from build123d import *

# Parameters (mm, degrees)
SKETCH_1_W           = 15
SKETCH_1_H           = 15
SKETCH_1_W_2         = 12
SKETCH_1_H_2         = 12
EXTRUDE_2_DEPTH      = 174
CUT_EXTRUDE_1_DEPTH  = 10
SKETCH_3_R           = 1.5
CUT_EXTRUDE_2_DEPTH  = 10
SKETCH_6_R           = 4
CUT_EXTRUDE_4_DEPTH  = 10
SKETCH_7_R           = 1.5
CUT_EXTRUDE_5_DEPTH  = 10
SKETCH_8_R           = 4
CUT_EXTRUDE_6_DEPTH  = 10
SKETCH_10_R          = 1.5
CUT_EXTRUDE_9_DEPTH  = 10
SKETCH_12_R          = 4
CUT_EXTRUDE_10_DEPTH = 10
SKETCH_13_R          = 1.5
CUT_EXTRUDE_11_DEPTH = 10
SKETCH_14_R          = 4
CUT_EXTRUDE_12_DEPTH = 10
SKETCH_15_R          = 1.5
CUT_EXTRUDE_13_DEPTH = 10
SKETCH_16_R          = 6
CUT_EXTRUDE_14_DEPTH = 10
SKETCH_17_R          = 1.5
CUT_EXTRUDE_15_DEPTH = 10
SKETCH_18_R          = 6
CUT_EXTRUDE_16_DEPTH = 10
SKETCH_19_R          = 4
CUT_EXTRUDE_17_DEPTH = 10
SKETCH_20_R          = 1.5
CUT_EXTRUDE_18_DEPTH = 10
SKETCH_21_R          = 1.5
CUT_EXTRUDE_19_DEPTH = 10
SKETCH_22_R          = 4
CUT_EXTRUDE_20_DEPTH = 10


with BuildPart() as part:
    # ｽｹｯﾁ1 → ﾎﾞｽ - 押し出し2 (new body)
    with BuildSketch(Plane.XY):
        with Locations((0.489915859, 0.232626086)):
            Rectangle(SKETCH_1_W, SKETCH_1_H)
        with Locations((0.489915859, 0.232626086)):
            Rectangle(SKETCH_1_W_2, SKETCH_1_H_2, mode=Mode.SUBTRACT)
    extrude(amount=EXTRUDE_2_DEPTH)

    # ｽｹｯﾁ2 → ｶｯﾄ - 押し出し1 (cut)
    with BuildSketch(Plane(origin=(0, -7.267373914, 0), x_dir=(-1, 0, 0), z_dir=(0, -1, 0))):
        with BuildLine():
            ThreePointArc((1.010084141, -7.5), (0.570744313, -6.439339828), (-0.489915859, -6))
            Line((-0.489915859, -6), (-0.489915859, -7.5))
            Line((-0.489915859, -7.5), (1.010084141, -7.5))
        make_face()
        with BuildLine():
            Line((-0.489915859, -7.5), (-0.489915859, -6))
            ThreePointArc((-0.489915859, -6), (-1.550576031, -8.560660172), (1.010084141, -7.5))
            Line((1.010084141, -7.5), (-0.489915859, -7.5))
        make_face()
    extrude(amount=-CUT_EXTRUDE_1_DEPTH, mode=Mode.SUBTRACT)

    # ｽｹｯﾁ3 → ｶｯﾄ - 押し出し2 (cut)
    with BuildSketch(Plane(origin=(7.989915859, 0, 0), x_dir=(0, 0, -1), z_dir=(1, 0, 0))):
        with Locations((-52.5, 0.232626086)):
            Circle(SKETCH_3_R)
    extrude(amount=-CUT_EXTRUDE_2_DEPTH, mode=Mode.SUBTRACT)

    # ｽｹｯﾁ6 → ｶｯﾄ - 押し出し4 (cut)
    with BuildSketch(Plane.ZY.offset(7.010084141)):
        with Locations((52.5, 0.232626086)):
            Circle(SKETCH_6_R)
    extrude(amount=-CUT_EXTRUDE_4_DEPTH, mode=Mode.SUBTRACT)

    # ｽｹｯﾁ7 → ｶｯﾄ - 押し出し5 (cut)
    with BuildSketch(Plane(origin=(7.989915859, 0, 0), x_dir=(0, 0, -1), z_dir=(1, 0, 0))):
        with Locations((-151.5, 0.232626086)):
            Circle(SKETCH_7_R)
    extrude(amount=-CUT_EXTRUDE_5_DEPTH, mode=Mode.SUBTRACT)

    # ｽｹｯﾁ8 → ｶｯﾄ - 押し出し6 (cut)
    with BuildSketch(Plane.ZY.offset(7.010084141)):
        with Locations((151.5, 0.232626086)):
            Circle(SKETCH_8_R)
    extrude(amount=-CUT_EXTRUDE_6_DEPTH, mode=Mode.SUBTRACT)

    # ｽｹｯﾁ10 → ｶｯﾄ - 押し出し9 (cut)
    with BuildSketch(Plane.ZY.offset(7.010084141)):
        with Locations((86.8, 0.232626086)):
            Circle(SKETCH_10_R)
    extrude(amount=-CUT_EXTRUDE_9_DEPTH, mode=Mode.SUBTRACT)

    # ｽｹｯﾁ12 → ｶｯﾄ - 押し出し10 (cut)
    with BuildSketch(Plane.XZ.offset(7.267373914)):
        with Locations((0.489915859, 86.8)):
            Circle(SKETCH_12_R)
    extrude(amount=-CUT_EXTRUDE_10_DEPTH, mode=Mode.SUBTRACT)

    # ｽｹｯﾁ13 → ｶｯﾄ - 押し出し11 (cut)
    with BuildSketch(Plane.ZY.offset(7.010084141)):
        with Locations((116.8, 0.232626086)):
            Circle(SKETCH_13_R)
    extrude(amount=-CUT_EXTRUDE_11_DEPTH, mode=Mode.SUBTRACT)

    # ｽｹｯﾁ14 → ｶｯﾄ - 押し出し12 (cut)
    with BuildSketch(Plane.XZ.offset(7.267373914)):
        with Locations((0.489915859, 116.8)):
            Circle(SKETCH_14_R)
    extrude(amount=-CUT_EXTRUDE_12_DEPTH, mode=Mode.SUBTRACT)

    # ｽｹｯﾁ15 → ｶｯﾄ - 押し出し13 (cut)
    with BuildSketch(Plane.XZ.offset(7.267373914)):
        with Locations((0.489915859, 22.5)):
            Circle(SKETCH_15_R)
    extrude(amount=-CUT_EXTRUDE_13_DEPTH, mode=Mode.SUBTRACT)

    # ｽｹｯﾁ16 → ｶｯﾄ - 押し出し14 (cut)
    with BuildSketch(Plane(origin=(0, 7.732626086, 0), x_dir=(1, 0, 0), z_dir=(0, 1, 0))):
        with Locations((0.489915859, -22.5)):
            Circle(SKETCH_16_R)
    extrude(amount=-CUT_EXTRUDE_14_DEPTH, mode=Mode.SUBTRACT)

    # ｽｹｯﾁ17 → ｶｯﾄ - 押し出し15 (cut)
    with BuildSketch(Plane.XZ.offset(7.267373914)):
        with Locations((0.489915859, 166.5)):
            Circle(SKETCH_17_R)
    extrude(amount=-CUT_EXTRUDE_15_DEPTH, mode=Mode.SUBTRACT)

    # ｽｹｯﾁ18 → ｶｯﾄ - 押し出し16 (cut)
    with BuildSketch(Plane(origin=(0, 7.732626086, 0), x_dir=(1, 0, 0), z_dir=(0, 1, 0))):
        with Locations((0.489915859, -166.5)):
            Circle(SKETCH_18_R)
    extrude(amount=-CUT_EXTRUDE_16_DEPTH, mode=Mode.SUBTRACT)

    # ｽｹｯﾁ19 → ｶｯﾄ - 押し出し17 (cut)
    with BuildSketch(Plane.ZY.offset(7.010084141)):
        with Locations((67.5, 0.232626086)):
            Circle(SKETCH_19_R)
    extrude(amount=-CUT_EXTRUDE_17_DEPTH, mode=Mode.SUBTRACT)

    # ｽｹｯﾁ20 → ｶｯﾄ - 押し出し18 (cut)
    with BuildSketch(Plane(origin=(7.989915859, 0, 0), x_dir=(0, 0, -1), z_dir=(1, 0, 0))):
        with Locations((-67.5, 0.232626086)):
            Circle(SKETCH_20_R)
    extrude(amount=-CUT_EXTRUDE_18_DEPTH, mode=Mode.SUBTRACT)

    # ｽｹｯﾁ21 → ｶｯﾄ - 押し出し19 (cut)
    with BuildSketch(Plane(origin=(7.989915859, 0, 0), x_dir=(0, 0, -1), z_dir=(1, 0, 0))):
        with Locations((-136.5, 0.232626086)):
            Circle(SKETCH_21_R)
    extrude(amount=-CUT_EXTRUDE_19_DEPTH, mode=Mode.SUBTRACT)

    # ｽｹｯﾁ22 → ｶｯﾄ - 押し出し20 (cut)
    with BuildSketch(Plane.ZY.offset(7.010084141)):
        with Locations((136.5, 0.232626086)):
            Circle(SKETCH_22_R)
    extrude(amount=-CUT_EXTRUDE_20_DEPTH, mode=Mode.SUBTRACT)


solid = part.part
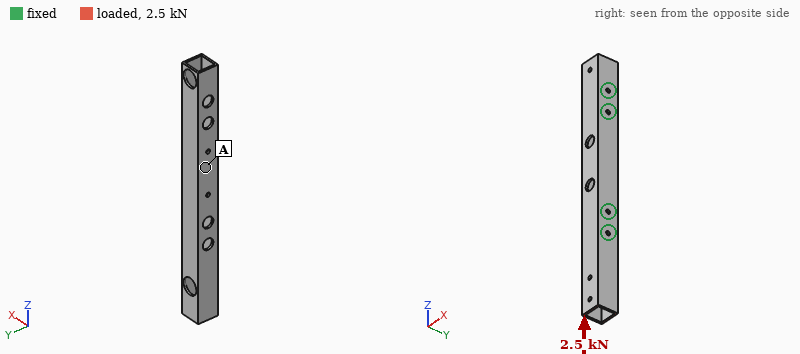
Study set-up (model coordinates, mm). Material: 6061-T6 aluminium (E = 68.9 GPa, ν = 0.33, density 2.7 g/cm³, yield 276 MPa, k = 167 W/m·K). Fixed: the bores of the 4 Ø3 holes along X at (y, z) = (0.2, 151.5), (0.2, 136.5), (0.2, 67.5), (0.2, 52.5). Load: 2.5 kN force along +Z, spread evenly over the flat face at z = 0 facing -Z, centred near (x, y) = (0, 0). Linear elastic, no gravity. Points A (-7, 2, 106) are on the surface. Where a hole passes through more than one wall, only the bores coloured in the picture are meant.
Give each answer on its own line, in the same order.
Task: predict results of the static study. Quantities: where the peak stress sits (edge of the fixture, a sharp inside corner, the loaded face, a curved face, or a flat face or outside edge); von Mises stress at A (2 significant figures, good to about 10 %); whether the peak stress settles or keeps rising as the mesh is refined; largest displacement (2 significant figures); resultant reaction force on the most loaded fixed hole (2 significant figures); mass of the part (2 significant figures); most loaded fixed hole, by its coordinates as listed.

edge of the fixture
14 MPa
keeps rising
0.15 mm
1.1 kN
36 g
(0.2, 52.5)
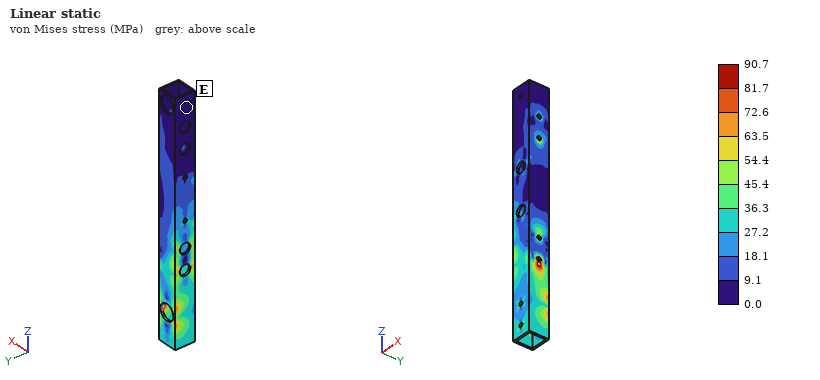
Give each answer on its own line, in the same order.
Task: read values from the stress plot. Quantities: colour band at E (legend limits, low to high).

0.0 to 9.1 MPa
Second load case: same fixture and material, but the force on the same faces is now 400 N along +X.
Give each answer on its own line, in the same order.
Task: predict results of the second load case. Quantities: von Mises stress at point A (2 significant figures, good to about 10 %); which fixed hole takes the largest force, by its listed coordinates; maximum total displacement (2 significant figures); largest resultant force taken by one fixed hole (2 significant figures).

19 MPa
(0.2, 52.5)
0.40 mm
1.2 kN
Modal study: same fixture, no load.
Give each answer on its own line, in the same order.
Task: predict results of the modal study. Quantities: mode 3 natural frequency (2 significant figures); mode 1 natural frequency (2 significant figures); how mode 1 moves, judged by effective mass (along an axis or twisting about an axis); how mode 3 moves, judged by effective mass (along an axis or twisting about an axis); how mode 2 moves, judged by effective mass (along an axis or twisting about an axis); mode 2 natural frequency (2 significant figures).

3200 Hz
2100 Hz
along Y
twisting about X
along X
2600 Hz
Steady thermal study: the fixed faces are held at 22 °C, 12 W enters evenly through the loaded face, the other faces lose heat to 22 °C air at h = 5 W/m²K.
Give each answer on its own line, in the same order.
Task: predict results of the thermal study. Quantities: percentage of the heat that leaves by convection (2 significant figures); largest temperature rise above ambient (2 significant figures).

8.4 %
58 K
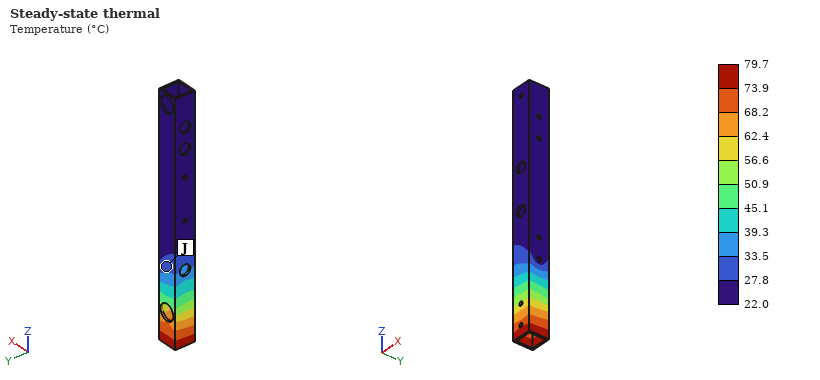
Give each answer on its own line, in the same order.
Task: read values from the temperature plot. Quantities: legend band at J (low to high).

27.8 to 33.5 °C
